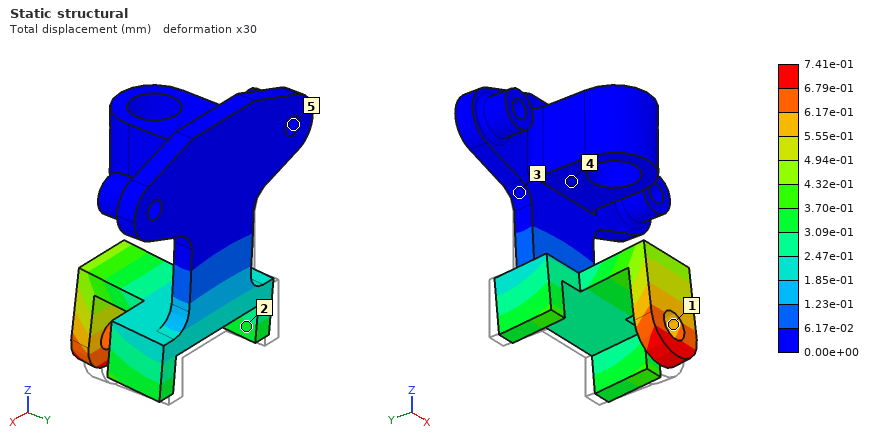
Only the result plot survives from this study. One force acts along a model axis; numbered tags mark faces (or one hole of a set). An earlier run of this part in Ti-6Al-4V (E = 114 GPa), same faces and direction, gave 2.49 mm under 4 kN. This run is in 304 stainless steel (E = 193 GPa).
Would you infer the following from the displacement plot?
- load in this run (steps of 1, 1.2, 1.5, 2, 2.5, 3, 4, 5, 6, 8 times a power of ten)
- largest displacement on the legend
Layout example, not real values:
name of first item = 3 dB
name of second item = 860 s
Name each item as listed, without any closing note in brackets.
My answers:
load in this run = 2 kN
largest displacement on the legend = 7.41e-01 mm
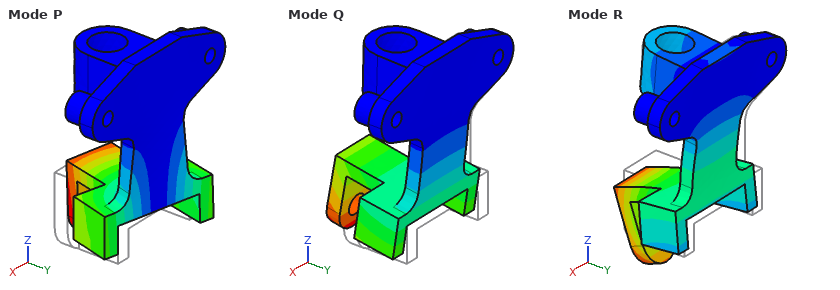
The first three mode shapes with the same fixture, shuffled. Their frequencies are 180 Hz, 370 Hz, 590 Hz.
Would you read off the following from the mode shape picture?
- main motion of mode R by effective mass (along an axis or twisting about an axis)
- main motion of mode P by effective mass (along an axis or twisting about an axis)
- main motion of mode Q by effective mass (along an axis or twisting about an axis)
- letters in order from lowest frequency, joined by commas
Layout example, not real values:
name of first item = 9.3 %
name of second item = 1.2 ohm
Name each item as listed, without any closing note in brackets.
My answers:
main motion of mode R by effective mass = along Y
main motion of mode P by effective mass = along X
main motion of mode Q by effective mass = along Y
letters in order from lowest frequency, joined by commas = Q, P, R
